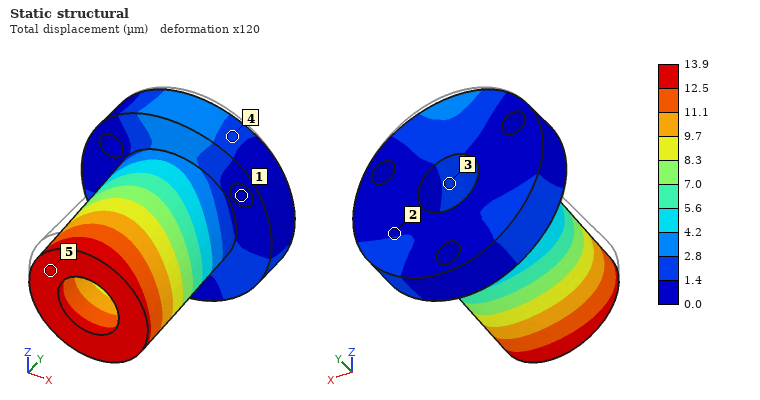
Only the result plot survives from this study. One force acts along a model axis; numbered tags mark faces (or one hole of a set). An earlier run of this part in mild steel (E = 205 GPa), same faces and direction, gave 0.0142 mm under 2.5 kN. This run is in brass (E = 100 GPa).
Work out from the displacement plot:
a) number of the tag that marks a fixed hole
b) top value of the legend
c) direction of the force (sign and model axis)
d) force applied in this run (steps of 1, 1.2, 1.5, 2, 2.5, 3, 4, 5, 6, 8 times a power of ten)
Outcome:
1
13.9 µm
-Z
1.2 kN
